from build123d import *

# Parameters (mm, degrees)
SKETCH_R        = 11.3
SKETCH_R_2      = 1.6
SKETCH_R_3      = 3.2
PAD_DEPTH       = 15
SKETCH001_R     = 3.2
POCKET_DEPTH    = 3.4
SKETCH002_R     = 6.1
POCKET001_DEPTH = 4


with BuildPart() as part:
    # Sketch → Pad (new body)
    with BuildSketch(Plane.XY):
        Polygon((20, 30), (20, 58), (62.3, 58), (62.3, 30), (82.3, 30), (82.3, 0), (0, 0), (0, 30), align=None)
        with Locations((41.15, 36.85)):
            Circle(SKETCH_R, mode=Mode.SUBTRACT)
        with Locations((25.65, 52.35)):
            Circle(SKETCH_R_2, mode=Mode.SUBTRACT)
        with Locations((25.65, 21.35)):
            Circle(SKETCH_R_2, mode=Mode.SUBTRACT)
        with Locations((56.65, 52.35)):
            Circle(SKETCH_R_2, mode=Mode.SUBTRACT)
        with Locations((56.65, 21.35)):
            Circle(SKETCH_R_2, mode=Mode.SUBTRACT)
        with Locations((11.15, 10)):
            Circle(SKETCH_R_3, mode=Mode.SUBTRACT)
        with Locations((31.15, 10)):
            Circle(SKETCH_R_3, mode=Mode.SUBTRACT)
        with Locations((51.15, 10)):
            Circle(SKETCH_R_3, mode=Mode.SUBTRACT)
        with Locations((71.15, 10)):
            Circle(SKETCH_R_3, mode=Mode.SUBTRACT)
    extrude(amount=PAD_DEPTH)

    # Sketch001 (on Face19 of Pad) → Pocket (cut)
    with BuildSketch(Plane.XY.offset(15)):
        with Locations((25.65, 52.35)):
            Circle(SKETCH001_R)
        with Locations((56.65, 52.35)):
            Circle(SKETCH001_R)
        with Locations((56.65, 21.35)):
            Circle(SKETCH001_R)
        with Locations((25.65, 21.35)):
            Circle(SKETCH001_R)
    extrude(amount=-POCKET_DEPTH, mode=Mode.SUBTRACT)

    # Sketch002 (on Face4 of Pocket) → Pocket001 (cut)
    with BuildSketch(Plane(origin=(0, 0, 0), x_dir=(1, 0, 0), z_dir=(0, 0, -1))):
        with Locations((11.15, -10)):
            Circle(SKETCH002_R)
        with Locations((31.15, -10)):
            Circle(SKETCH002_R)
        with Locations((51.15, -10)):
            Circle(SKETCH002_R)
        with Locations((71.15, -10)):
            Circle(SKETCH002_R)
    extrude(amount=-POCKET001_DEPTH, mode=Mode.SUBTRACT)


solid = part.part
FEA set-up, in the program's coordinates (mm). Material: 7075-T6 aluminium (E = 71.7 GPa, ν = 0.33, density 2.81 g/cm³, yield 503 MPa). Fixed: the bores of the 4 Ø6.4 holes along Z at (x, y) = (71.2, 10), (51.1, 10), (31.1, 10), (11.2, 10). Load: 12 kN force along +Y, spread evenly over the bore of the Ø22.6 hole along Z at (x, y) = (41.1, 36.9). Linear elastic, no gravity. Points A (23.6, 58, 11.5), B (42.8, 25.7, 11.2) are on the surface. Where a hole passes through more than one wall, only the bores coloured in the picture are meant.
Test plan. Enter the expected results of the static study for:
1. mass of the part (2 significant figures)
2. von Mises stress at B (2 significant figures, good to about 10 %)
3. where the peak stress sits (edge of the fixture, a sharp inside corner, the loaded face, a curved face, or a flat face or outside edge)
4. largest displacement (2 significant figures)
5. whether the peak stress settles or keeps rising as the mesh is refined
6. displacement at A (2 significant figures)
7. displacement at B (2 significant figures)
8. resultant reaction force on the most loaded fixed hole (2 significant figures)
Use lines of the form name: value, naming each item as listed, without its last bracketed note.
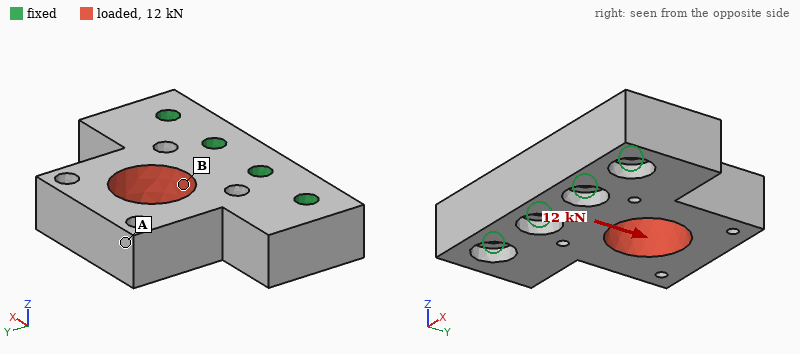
mass of the part: 130 g
von Mises stress at B: 12 MPa
where the peak stress sits: edge of the fixture
largest displacement: 20 µm
whether the peak stress settles or keeps rising as the mesh is refined: keeps rising
displacement at A: 12 µm
displacement at B: 3.9 µm
resultant reaction force on the most loaded fixed hole: 3.9 kN
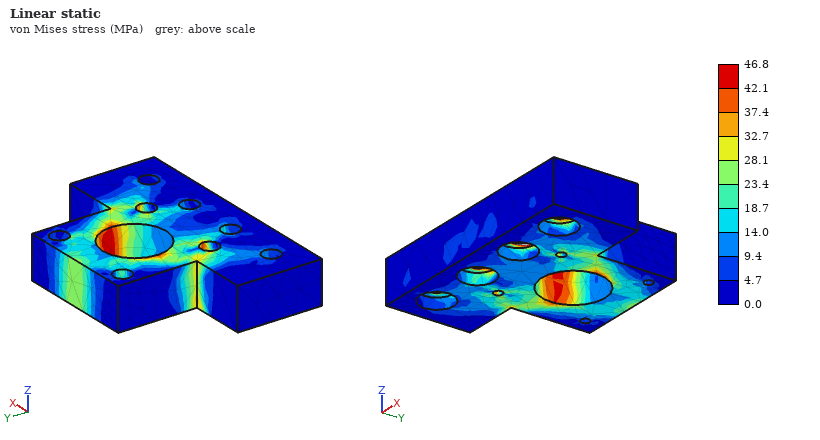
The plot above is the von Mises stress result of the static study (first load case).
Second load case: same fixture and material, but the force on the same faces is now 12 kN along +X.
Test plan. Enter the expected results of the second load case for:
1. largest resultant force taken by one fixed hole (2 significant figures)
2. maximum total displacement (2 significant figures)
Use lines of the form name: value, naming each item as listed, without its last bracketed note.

largest resultant force taken by one fixed hole: 5.6 kN
maximum total displacement: 55 µm
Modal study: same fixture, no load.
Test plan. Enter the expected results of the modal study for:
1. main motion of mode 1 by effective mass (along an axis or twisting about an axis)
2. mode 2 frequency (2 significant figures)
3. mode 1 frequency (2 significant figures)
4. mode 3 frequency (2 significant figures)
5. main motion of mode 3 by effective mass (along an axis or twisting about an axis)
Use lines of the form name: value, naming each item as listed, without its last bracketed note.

main motion of mode 1 by effective mass: along Z
mode 2 frequency: 10 kHz
mode 1 frequency: 4900 Hz
mode 3 frequency: 11 kHz
main motion of mode 3 by effective mass: along X
